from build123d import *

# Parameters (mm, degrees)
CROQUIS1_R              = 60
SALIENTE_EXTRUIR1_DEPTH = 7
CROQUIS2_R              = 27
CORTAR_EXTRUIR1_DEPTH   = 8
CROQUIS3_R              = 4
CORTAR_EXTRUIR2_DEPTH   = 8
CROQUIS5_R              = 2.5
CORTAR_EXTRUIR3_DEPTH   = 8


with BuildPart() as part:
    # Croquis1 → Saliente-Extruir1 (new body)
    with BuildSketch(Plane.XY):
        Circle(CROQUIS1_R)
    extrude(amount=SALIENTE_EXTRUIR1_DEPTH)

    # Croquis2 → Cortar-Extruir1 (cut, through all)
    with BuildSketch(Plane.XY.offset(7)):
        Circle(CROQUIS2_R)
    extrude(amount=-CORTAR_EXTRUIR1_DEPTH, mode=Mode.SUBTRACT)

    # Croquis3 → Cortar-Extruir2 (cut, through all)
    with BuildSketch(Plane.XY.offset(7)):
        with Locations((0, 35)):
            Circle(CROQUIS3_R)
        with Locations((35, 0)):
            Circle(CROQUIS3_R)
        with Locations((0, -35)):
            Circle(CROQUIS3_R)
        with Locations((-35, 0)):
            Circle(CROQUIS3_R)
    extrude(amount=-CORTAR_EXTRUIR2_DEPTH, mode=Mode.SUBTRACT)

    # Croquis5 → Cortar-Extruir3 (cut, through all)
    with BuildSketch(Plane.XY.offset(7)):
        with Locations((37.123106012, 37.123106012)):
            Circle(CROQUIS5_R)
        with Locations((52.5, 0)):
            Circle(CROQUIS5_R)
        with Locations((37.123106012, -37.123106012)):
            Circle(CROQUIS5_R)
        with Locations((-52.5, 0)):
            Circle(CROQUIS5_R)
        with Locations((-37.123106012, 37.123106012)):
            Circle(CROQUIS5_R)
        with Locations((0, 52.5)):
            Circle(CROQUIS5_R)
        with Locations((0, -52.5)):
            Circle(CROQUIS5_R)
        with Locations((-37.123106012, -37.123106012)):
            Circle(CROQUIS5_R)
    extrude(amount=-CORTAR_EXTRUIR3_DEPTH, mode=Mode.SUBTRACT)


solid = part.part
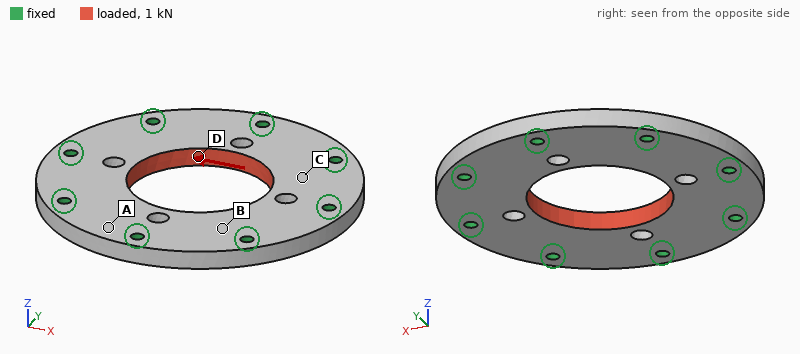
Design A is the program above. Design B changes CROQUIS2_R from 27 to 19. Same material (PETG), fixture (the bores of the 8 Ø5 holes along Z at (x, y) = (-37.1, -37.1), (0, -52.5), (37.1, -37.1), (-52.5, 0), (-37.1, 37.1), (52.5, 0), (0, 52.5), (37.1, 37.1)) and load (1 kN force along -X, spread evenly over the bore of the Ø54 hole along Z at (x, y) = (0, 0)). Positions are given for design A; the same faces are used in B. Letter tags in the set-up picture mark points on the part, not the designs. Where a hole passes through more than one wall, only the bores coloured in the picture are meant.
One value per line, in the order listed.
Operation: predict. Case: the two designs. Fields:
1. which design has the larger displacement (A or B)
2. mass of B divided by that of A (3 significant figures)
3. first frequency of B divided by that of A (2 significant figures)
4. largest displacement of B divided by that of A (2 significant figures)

B
1.13
0.72
1.2
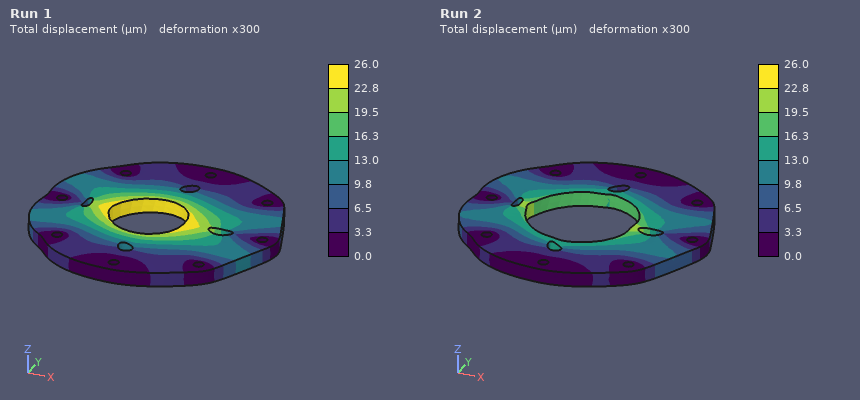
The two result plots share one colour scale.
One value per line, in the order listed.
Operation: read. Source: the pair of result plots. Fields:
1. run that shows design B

Run 1
